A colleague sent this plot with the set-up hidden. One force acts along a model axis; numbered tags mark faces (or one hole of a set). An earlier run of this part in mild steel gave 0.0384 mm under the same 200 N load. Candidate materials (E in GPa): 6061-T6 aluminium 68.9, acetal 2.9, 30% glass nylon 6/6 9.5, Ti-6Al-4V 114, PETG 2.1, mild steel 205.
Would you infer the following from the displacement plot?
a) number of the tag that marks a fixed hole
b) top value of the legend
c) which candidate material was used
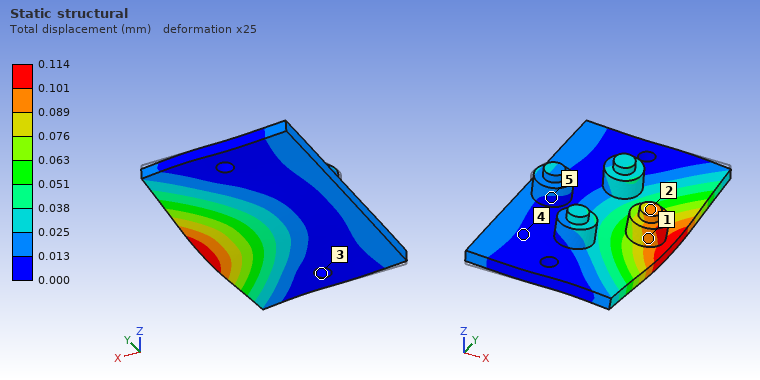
3
0.114 mm
6061-T6 aluminium
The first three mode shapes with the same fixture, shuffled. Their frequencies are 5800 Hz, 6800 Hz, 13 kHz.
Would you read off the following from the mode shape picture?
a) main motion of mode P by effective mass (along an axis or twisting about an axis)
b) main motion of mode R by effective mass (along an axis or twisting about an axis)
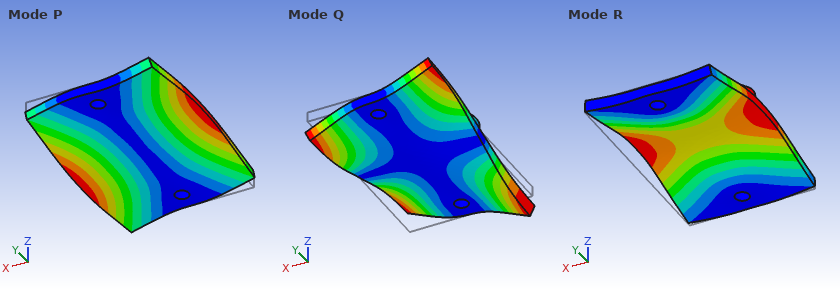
twisting about Y
along Z
